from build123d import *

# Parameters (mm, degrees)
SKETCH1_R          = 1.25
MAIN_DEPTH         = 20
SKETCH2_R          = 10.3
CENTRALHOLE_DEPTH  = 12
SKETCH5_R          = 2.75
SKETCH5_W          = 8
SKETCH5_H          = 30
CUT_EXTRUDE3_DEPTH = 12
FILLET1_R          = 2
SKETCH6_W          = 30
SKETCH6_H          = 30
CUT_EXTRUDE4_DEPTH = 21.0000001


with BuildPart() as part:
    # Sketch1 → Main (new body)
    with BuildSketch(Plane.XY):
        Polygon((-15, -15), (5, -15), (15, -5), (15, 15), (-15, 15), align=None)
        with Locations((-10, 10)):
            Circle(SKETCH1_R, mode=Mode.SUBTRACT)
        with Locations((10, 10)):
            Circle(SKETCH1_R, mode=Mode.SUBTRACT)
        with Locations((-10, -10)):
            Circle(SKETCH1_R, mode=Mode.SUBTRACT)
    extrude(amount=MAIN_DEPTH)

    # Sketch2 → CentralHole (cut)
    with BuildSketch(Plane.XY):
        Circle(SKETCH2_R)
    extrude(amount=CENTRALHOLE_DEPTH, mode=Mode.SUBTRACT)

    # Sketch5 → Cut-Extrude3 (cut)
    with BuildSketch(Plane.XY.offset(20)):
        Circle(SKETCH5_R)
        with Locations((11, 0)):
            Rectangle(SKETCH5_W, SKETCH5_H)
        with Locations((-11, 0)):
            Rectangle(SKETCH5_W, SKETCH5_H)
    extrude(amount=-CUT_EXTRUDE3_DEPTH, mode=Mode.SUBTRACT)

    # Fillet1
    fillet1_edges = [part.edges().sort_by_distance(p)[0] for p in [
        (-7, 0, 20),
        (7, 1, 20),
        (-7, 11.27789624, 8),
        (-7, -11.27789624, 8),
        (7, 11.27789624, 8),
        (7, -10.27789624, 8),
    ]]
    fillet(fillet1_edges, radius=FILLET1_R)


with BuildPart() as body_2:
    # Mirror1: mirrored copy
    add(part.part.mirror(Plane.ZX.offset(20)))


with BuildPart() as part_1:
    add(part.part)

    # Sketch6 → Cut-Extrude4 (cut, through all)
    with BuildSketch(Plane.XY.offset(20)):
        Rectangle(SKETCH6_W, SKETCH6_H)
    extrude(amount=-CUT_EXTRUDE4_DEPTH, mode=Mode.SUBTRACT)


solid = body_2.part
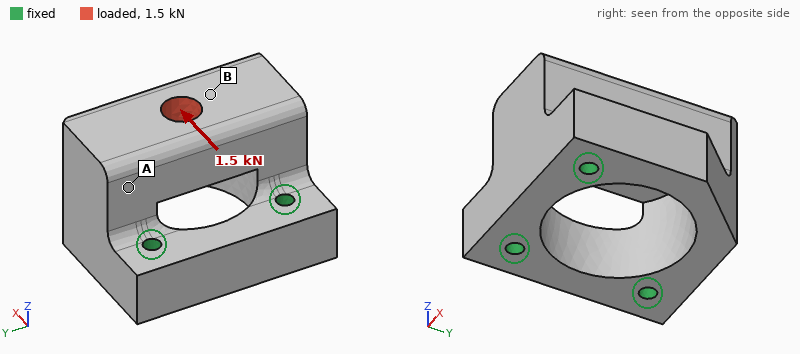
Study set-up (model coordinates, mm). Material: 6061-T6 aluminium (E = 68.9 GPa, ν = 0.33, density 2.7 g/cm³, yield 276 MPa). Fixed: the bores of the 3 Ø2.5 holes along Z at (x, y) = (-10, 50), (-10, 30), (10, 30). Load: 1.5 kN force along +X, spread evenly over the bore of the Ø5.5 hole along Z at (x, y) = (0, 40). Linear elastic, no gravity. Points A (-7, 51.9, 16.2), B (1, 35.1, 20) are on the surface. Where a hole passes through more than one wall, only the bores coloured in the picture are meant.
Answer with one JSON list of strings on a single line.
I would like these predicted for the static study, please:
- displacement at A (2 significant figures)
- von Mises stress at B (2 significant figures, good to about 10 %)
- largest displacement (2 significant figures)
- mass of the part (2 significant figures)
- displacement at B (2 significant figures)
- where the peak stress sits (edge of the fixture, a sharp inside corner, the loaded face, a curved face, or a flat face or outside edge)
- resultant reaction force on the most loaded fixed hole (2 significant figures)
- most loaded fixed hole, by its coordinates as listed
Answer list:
["16 µm", "28 MPa", "25 µm", "21 g", "17 µm", "edge of the fixture", "880 N", "(10, 30)"]
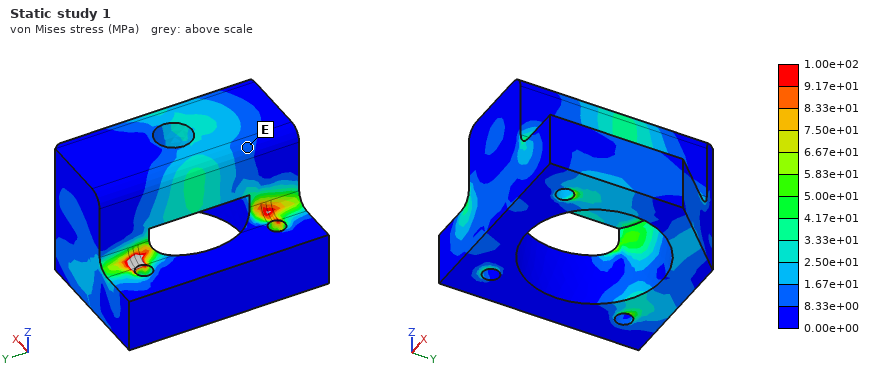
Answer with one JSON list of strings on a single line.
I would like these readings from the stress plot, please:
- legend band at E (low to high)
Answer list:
["8.33e+00 to 1.67e+01 MPa"]
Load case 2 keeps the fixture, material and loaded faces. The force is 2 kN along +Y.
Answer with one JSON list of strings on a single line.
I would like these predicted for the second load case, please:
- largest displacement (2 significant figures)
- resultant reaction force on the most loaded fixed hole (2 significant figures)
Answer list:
["29 µm", "870 N"]
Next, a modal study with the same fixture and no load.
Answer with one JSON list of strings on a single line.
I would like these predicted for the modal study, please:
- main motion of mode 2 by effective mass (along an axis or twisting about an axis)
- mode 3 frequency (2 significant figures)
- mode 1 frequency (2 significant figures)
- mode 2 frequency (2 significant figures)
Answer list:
["along Y", "26 kHz", "13 kHz", "17 kHz"]
